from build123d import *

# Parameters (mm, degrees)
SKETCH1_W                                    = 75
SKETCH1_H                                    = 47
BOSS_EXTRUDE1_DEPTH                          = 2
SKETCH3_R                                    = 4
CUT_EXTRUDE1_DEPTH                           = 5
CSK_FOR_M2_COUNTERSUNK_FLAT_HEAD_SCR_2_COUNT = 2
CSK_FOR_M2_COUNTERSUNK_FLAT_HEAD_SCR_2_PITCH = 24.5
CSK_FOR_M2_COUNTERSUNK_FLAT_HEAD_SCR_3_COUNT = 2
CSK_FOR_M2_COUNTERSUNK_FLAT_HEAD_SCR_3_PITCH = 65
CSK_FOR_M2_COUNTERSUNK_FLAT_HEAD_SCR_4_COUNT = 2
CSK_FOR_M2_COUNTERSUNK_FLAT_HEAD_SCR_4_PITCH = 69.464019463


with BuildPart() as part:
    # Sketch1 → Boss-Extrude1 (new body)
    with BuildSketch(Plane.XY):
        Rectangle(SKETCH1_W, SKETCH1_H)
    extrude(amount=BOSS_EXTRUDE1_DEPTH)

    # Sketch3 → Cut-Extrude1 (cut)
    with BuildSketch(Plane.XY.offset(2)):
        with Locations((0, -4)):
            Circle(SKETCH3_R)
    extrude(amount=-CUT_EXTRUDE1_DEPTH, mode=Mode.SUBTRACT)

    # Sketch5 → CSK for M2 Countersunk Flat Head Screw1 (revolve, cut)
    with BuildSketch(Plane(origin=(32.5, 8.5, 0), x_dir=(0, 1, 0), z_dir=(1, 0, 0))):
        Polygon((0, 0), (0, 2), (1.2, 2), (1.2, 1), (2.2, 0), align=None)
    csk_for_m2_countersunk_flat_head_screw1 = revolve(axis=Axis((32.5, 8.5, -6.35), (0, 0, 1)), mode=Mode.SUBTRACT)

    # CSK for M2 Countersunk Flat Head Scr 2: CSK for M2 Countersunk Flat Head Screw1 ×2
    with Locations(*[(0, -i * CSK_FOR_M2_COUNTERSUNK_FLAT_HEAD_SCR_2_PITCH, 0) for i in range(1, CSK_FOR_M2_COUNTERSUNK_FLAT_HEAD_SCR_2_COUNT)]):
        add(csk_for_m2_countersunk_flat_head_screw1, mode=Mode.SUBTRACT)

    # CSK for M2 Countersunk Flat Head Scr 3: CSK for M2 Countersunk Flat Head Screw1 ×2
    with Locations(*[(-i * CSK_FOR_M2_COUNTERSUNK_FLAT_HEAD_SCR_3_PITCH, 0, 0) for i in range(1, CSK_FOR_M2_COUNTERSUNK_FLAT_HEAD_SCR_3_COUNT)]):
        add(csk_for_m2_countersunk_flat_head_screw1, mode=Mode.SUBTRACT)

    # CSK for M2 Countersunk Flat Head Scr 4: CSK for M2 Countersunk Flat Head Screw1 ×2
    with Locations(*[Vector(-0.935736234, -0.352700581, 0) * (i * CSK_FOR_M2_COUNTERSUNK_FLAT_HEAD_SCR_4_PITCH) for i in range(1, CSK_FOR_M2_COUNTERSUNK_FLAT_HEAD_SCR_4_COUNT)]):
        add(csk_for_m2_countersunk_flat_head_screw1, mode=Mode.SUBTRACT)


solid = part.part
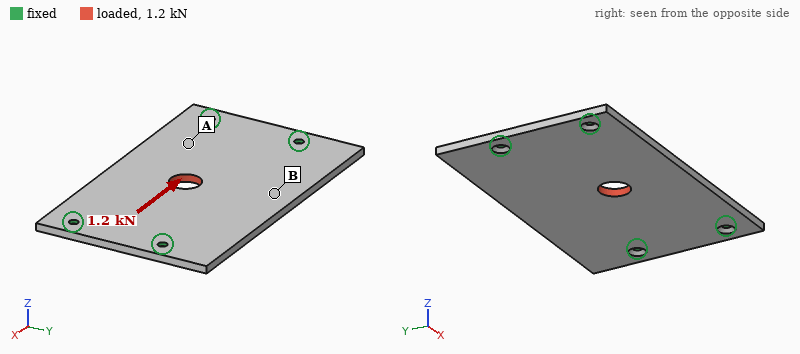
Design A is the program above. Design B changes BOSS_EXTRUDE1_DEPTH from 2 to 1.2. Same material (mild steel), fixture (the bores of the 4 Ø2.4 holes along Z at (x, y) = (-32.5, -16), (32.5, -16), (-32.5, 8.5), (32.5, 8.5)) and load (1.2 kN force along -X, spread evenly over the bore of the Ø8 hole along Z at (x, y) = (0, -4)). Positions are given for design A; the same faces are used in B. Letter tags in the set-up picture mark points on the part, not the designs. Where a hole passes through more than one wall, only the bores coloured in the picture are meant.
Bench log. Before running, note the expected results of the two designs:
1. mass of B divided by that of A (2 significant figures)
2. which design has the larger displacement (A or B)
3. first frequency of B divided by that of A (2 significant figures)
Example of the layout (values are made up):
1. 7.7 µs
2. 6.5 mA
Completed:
1. 0.60
2. B
3. 0.59
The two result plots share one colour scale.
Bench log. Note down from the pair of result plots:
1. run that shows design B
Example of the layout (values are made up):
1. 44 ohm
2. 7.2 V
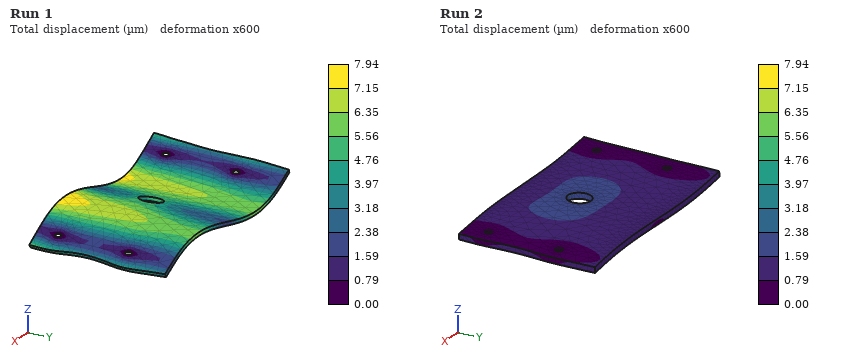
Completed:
1. Run 1
